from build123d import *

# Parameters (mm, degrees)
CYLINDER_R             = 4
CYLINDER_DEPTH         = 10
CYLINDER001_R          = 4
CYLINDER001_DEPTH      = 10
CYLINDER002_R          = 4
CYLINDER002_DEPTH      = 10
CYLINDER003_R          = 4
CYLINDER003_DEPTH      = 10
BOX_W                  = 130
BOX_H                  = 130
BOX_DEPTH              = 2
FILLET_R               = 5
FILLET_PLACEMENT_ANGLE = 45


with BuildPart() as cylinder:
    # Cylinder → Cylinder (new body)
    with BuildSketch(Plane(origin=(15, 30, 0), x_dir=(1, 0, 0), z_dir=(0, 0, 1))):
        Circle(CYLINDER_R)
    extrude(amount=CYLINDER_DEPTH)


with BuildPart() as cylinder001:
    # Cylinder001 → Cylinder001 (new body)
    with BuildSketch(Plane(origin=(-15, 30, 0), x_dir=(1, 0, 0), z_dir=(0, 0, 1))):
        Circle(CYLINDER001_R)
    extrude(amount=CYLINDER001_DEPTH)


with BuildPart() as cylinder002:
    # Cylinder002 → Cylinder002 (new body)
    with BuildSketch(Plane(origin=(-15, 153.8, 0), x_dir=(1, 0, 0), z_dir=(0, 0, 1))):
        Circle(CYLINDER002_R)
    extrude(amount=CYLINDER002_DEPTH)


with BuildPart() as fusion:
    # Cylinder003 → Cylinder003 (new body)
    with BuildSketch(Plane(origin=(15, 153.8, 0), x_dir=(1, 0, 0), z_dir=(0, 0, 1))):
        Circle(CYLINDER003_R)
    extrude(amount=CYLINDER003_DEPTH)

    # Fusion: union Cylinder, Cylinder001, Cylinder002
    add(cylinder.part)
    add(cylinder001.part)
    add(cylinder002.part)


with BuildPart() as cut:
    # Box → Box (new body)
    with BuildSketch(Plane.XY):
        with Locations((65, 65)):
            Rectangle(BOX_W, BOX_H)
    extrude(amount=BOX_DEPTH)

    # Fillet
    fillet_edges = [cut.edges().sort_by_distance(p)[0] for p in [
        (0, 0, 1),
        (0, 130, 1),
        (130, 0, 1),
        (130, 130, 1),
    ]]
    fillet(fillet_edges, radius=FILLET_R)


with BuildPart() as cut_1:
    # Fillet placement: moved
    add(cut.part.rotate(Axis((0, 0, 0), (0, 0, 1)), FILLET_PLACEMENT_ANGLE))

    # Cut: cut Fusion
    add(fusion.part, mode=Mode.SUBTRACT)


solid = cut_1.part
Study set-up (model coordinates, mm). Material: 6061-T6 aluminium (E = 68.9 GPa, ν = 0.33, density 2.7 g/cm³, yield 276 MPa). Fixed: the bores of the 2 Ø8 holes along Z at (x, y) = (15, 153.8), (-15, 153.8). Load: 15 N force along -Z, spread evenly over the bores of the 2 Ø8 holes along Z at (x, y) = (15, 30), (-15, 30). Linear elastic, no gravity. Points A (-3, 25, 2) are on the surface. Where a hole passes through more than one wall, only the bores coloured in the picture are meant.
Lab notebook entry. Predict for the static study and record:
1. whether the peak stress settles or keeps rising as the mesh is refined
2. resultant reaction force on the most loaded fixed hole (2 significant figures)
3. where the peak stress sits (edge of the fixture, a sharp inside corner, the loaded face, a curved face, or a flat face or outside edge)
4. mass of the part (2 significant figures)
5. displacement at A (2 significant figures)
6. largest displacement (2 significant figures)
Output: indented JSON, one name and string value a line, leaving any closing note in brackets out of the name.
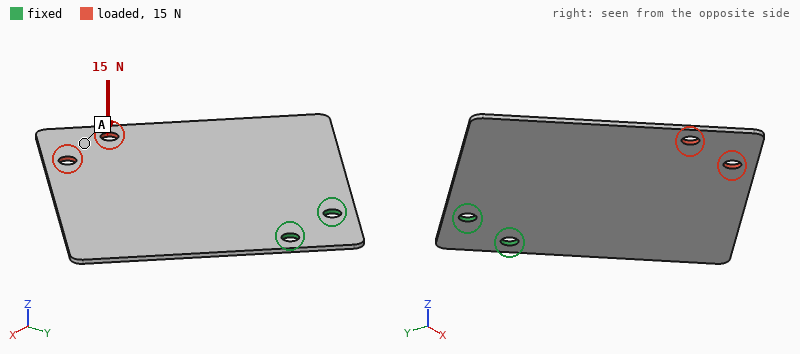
{
  "whether the peak stress settles or keeps rising as the mesh is refined": "keeps rising",
  "resultant reaction force on the most loaded fixed hole": "7.6 N",
  "where the peak stress sits": "edge of the fixture",
  "mass of the part": "90 g",
  "displacement at A": "2.1 mm",
  "largest displacement": "2.6 mm"
}
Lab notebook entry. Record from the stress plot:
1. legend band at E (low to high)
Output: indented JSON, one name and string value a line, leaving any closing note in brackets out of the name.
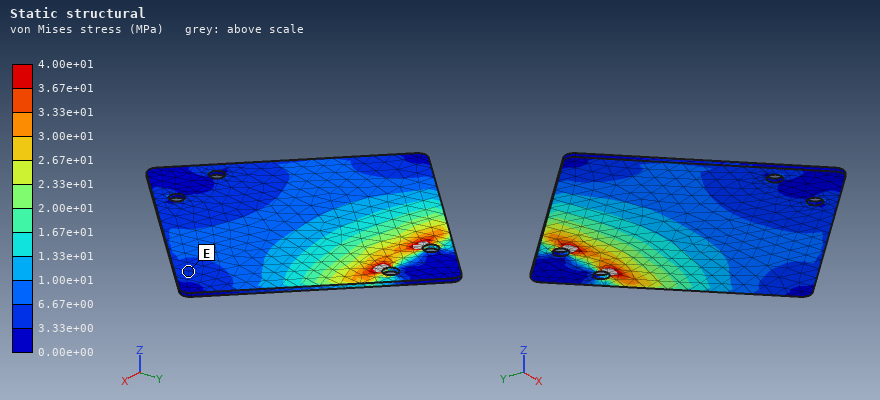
{
  "legend band at E": "3.33e+00 to 6.67e+00 MPa"
}
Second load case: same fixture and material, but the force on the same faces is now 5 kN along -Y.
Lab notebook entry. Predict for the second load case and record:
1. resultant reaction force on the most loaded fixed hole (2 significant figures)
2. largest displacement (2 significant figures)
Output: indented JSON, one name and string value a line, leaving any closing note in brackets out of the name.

{
  "resultant reaction force on the most loaded fixed hole": "2.5 kN",
  "largest displacement": "71 µm"
}
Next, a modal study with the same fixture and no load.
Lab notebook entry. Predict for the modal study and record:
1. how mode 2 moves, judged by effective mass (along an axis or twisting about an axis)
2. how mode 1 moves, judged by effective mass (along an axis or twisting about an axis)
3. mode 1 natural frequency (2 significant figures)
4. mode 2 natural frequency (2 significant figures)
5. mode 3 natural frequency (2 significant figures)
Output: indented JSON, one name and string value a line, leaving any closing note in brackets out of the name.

{
  "how mode 2 moves, judged by effective mass": "twisting about Y",
  "how mode 1 moves, judged by effective mass": "along Z",
  "mode 1 natural frequency": "91 Hz",
  "mode 2 natural frequency": "190 Hz",
  "mode 3 natural frequency": "370 Hz"
}
